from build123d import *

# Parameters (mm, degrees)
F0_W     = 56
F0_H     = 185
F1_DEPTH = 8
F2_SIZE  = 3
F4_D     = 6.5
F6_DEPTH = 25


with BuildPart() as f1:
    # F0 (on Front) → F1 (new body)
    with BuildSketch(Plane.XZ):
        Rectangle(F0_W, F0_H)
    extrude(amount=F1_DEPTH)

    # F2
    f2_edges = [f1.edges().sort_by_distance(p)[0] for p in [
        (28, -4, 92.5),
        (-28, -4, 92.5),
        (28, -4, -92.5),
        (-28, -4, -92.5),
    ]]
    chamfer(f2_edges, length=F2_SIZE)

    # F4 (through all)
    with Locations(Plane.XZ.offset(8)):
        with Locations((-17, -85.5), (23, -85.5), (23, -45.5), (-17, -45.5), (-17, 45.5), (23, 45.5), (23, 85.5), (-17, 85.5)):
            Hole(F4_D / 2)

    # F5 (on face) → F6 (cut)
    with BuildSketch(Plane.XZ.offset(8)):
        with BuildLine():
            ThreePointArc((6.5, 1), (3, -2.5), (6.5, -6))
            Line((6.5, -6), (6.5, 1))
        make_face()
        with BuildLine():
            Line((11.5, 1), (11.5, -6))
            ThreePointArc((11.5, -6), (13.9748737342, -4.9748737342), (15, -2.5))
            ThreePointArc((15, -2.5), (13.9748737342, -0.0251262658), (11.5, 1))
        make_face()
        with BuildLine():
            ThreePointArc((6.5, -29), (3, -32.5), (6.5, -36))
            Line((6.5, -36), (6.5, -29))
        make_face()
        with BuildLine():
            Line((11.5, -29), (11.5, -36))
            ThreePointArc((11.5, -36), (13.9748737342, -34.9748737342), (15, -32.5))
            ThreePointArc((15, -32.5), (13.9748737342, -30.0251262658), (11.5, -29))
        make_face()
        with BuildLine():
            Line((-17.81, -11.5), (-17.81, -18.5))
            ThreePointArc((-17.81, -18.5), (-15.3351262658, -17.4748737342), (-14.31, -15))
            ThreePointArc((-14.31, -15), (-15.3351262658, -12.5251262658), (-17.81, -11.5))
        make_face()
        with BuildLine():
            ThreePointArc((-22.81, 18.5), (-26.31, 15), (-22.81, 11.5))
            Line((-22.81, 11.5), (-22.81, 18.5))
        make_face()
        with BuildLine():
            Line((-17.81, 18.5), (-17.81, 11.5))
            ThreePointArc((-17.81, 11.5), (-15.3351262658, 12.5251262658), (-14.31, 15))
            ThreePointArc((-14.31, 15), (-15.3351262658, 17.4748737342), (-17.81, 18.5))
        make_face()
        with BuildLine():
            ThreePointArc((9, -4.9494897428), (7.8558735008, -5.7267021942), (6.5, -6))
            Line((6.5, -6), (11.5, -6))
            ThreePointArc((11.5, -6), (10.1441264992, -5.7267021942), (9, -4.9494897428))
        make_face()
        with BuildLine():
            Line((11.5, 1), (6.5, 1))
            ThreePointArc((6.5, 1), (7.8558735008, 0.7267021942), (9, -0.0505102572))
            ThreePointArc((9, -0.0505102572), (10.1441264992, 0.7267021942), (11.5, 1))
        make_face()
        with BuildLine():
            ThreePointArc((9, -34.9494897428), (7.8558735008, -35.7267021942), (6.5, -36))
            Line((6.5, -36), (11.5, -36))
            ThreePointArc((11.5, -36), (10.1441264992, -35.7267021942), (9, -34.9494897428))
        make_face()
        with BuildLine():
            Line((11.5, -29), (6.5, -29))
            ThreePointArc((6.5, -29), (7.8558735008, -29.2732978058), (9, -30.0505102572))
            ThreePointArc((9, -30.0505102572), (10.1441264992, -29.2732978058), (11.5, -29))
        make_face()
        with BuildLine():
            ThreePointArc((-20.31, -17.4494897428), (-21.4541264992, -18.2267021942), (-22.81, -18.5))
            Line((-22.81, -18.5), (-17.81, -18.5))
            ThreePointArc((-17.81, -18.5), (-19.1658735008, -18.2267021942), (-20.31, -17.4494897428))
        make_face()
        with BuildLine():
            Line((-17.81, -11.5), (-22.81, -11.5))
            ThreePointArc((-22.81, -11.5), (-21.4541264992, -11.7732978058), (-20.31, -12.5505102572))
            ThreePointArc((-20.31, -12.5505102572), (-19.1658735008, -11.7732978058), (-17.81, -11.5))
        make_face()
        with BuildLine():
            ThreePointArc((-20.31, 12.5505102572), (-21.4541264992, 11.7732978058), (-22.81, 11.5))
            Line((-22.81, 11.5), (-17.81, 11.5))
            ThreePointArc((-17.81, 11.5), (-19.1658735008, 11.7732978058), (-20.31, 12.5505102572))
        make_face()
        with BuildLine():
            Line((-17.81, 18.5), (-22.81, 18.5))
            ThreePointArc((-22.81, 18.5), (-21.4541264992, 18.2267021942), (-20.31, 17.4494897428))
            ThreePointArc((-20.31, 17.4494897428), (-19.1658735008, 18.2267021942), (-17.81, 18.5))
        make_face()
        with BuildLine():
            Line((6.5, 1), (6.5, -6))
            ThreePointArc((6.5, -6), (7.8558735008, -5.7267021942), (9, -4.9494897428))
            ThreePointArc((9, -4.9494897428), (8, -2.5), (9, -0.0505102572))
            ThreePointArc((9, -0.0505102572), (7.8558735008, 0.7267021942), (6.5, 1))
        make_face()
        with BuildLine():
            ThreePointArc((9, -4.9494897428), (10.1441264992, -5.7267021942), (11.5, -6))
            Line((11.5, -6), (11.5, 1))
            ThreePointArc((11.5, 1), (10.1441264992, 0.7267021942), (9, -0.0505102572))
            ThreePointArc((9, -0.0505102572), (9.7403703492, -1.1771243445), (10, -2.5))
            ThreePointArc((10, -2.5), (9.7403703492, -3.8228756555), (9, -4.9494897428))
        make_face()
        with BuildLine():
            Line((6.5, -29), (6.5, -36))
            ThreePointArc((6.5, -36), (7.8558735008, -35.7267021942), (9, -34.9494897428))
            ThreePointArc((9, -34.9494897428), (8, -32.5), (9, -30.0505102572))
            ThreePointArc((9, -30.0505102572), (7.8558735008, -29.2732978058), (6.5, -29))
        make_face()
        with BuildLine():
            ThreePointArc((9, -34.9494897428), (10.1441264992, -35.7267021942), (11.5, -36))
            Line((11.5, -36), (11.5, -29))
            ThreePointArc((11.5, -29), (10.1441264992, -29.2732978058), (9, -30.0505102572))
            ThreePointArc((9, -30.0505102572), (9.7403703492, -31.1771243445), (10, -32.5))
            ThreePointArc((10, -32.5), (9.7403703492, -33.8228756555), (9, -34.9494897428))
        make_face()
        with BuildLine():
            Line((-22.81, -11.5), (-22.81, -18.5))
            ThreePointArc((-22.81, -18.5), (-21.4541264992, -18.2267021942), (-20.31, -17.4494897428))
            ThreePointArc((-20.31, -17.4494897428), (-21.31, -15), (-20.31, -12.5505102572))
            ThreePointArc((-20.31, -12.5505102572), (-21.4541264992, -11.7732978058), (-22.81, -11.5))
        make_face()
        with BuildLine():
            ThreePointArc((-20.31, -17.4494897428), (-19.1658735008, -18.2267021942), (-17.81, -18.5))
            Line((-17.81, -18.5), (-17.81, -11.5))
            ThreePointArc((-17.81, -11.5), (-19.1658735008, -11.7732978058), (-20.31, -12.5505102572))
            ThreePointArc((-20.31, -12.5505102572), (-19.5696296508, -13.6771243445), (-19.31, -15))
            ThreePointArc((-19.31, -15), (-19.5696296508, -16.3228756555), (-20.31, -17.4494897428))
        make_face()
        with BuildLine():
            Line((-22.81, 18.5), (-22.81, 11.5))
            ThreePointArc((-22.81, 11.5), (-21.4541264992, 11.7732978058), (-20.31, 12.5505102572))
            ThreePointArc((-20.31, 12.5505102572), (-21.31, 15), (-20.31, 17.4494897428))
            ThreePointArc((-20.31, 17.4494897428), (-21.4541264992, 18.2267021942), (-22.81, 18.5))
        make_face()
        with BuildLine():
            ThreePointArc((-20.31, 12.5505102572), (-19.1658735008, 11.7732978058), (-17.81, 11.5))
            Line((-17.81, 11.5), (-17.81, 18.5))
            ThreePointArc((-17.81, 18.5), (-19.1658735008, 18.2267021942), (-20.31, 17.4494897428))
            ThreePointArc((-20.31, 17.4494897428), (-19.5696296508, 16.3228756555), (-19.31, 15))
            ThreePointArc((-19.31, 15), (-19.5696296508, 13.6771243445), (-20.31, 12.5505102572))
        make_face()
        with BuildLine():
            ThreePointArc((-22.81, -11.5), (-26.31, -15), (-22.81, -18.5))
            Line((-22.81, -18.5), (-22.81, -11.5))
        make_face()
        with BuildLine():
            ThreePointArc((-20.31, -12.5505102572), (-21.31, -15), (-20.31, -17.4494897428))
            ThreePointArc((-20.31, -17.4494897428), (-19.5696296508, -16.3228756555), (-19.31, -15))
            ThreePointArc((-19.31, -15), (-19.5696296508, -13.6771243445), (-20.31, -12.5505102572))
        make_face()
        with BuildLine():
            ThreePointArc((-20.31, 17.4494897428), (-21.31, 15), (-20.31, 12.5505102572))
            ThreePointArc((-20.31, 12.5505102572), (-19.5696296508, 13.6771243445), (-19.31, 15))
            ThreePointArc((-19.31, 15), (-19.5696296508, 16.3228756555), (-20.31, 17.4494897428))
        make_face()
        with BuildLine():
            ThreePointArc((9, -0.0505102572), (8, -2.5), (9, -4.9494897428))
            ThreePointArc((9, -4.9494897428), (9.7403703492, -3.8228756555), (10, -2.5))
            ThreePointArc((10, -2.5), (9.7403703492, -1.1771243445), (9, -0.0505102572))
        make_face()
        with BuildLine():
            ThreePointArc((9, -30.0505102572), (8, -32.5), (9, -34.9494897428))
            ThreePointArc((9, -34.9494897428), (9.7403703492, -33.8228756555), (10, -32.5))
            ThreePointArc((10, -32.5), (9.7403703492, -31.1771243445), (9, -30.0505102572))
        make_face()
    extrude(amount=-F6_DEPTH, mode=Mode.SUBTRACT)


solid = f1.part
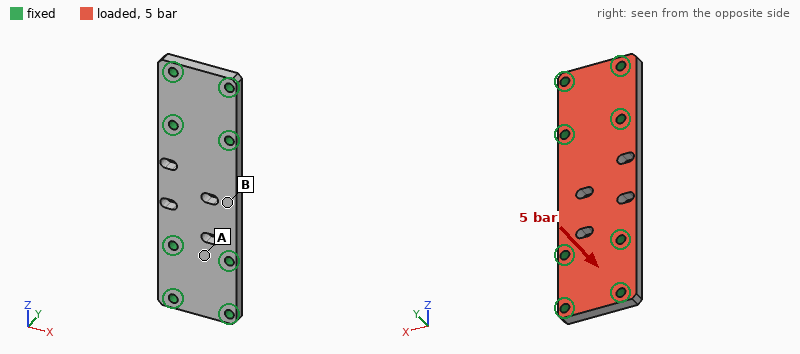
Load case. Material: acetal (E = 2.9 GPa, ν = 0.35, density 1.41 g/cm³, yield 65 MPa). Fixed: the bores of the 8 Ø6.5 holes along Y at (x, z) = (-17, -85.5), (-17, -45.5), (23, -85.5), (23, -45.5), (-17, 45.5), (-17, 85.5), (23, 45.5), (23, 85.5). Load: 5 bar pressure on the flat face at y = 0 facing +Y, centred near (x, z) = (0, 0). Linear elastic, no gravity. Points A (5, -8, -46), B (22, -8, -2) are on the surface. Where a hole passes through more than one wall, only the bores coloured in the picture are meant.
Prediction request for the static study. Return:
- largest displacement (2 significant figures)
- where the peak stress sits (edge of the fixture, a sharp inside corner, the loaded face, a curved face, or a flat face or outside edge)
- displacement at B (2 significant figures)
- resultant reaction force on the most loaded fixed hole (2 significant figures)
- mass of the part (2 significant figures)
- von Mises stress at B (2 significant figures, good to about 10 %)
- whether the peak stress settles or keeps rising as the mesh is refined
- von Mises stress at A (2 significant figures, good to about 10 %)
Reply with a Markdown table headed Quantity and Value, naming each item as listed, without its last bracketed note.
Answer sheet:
| Quantity | Value |
|---|---|
| largest displacement | 0.84 mm |
| where the peak stress sits | edge of the fixture |
| displacement at B | 0.82 mm |
| resultant reaction force on the most loaded fixed hole | 1.0 kN |
| mass of the part | 110 g |
| von Mises stress at B | 19 MPa |
| whether the peak stress settles or keeps rising as the mesh is refined | keeps rising |
| von Mises stress at A | 9.4 MPa |
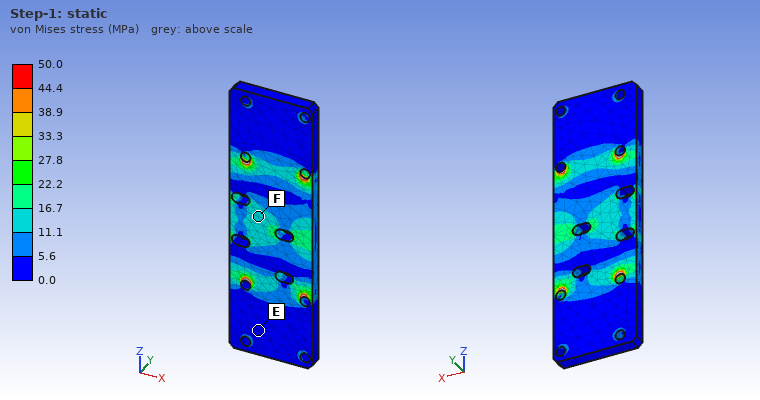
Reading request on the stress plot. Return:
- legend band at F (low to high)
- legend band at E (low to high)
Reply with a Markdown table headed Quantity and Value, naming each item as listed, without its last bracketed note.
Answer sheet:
| Quantity | Value |
|---|---|
| legend band at F | 11.1 to 16.7 MPa |
| legend band at E | 0.0 to 5.6 MPa |
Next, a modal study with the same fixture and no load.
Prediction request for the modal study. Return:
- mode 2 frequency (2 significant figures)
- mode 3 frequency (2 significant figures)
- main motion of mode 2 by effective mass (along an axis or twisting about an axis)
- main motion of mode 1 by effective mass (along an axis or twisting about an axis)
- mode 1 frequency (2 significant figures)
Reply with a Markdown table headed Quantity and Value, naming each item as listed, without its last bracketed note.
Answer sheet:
| Quantity | Value |
|---|---|
| mode 2 frequency | 2000 Hz |
| mode 3 frequency | 3300 Hz |
| main motion of mode 2 by effective mass | twisting about Z |
| main motion of mode 1 by effective mass | along Y |
| mode 1 frequency | 1300 Hz |
